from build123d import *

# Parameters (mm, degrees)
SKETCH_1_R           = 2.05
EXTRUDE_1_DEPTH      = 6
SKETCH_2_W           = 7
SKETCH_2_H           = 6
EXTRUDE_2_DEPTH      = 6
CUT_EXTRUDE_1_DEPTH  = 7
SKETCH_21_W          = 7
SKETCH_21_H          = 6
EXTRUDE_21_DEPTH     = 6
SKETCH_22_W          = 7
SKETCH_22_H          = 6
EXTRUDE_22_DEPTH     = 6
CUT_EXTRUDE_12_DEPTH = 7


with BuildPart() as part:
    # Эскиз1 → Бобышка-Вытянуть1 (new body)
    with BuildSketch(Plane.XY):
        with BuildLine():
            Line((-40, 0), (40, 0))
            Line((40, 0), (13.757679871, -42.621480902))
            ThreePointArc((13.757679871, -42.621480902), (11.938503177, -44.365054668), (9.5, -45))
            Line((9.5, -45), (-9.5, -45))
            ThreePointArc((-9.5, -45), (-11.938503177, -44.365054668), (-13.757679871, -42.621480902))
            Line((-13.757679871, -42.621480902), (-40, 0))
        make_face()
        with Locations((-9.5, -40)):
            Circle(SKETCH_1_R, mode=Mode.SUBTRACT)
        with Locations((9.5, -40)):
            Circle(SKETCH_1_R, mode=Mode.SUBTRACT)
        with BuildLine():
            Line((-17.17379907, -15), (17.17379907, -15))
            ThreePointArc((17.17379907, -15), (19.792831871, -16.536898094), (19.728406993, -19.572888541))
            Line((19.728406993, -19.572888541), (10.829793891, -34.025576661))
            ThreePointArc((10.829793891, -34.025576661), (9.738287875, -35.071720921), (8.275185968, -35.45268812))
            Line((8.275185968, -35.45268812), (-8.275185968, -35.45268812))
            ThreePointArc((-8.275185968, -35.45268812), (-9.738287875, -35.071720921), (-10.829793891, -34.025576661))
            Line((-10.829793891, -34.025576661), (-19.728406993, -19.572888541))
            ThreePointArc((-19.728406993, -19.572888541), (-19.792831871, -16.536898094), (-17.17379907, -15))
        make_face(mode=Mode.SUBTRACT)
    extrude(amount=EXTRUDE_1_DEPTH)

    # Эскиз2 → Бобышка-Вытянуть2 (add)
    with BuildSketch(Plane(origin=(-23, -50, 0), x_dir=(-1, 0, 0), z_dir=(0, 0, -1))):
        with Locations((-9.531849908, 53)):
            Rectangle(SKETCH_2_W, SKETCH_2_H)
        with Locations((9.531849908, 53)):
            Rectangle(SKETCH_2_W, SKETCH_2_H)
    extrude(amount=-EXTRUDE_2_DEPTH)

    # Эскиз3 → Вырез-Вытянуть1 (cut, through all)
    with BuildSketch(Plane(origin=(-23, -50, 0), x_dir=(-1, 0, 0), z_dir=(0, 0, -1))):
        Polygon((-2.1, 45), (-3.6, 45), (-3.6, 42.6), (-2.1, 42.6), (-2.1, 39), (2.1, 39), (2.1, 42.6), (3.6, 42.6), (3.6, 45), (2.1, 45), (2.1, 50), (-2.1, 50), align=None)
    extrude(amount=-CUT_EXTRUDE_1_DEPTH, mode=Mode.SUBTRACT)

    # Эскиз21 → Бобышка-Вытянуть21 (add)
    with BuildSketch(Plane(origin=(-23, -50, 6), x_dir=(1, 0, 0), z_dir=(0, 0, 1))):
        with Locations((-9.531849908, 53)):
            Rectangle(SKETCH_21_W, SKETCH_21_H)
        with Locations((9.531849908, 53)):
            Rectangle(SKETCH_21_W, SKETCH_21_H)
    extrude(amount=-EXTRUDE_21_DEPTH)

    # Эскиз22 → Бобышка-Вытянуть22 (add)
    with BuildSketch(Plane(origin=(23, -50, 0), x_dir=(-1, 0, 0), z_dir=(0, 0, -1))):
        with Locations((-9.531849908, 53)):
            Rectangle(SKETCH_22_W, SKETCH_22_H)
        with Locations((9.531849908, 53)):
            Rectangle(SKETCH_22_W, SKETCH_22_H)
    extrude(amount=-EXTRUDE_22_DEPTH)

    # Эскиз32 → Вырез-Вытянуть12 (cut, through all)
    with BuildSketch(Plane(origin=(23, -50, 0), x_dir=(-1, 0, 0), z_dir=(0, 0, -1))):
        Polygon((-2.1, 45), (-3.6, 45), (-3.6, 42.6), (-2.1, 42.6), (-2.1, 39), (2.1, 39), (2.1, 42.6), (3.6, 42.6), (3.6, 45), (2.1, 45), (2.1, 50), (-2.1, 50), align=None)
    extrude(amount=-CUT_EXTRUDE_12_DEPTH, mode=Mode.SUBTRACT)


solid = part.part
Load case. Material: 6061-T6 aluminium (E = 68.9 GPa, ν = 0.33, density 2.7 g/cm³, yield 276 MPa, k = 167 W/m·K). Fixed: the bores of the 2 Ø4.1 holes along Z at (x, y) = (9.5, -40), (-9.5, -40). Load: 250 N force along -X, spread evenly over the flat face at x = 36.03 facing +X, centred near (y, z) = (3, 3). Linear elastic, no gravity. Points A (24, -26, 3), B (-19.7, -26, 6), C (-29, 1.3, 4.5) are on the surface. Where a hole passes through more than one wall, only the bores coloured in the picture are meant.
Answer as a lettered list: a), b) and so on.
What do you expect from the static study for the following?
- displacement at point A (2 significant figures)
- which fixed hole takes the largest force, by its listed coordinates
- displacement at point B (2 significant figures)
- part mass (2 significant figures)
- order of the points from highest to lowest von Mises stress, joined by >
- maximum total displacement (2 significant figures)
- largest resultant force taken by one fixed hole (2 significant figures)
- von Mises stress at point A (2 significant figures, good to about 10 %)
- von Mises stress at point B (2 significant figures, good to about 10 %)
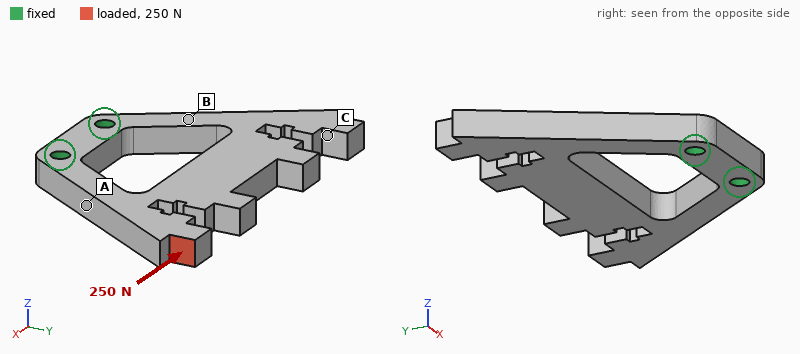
a) 0.045 mm
b) (-9.5, -40)
c) 0.040 mm
d) 28 g
e) A > B > C
f) 0.25 mm
g) 310 N
h) 31 MPa
i) 16 MPa
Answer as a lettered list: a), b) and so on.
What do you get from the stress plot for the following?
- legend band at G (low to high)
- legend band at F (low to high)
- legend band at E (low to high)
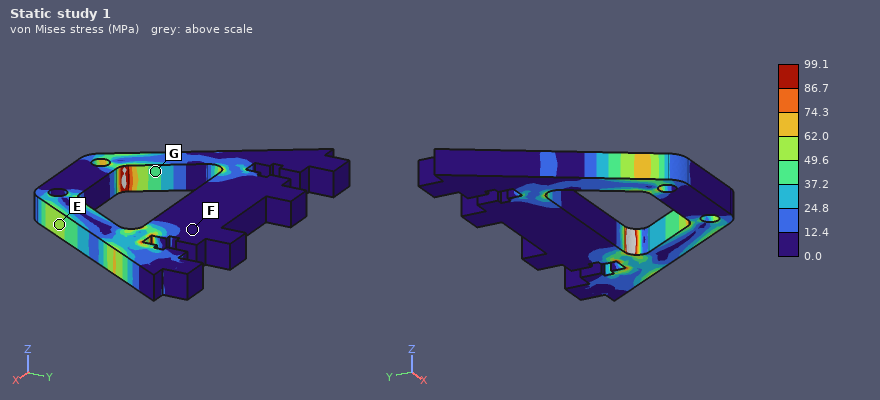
a) 37.2 to 49.6 MPa
b) 0.0 to 12.4 MPa
c) 49.6 to 62.0 MPa
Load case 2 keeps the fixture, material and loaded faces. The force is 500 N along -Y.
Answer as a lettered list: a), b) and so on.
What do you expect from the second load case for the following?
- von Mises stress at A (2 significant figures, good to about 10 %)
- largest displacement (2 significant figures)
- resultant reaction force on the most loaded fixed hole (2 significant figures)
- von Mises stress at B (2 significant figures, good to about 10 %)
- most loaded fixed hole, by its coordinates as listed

a) 46 MPa
b) 0.29 mm
c) 810 N
d) 18 MPa
e) (9.5, -40)
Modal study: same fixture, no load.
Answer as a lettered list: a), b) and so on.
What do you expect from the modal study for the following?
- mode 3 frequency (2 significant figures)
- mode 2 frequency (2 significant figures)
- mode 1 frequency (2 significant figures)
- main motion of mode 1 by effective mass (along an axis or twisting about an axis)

a) 1900 Hz
b) 1900 Hz
c) 1200 Hz
d) along Z
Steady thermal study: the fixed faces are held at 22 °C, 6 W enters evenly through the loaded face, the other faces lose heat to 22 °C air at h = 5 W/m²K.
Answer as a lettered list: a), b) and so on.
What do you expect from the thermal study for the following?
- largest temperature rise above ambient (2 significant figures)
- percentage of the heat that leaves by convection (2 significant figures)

a) 32 K
b) 4.6 %
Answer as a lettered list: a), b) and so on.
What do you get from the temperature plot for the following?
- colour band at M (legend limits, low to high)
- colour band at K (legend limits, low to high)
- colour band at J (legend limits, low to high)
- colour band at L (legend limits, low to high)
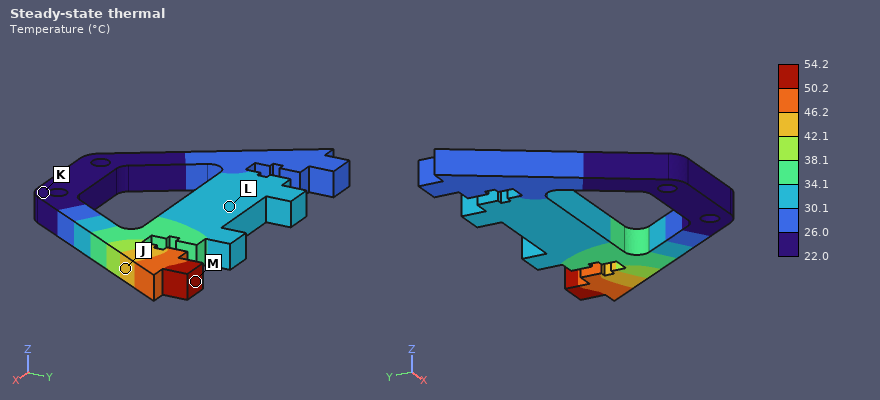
a) 50.2 to 54.2 °C
b) 22.0 to 26.0 °C
c) 42.1 to 46.2 °C
d) 30.1 to 34.1 °C
